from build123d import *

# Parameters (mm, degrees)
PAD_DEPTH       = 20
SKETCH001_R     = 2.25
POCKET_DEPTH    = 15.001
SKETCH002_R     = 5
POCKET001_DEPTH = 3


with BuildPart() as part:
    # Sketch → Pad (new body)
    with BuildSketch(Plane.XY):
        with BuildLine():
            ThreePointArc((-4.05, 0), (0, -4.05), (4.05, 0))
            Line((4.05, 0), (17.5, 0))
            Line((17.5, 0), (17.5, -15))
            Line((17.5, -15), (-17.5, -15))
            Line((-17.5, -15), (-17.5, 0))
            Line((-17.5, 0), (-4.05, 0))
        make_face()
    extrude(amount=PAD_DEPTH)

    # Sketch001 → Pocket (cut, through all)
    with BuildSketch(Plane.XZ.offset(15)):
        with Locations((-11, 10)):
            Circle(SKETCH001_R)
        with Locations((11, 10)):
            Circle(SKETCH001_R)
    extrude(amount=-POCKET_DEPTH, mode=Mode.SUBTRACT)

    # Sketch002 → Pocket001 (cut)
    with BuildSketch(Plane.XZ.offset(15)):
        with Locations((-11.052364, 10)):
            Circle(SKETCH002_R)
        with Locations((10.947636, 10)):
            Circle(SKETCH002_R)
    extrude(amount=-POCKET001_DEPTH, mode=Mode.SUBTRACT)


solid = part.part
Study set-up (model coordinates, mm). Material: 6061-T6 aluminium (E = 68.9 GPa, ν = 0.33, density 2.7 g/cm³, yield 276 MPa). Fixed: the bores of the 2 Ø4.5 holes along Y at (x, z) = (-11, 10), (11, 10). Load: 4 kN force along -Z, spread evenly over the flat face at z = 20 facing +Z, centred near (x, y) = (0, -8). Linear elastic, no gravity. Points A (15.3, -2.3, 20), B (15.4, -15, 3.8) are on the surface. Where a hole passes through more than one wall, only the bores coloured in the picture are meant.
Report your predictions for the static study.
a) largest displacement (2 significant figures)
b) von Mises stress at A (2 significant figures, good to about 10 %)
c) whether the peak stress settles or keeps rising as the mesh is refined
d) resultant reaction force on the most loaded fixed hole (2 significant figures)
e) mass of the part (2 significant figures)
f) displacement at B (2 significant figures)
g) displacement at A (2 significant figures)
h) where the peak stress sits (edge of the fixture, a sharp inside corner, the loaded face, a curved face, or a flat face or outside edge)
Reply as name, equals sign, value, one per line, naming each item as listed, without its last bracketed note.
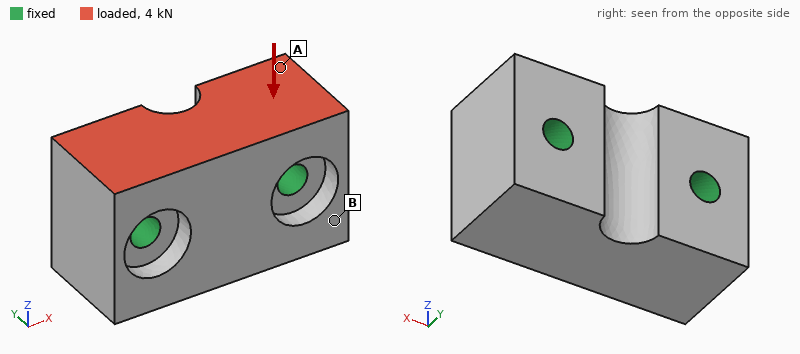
largest displacement = 3.6 µm
von Mises stress at A = 8.3 MPa
whether the peak stress settles or keeps rising as the mesh is refined = keeps rising
resultant reaction force on the most loaded fixed hole = 2.0 kN
mass of the part = 25 g
displacement at B = 0.88 µm
displacement at A = 1.2 µm
where the peak stress sits = edge of the fixture
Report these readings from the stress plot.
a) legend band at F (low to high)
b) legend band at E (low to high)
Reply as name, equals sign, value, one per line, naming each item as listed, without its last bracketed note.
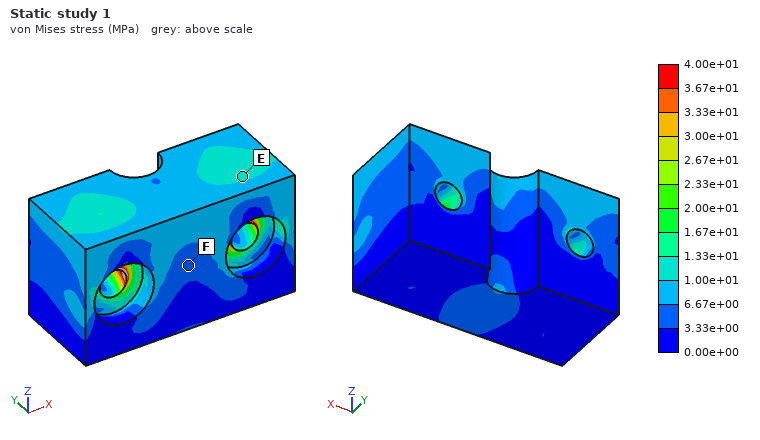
legend band at F = 3.33e+00 to 6.67e+00 MPa
legend band at E = 1.00e+01 to 1.33e+01 MPa
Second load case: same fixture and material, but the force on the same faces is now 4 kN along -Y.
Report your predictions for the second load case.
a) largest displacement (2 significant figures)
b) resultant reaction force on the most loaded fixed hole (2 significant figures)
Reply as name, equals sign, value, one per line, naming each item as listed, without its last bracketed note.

largest displacement = 12 µm
resultant reaction force on the most loaded fixed hole = 2.0 kN
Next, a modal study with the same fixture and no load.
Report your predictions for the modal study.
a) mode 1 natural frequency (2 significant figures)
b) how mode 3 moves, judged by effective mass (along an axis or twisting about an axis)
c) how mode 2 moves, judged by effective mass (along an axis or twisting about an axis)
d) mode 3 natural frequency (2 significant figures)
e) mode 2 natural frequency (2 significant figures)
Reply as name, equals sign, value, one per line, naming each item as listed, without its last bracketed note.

mode 1 natural frequency = 39 kHz
how mode 3 moves, judged by effective mass = twisting about Y
how mode 2 moves, judged by effective mass = along Y
mode 3 natural frequency = 52 kHz
mode 2 natural frequency = 48 kHz
